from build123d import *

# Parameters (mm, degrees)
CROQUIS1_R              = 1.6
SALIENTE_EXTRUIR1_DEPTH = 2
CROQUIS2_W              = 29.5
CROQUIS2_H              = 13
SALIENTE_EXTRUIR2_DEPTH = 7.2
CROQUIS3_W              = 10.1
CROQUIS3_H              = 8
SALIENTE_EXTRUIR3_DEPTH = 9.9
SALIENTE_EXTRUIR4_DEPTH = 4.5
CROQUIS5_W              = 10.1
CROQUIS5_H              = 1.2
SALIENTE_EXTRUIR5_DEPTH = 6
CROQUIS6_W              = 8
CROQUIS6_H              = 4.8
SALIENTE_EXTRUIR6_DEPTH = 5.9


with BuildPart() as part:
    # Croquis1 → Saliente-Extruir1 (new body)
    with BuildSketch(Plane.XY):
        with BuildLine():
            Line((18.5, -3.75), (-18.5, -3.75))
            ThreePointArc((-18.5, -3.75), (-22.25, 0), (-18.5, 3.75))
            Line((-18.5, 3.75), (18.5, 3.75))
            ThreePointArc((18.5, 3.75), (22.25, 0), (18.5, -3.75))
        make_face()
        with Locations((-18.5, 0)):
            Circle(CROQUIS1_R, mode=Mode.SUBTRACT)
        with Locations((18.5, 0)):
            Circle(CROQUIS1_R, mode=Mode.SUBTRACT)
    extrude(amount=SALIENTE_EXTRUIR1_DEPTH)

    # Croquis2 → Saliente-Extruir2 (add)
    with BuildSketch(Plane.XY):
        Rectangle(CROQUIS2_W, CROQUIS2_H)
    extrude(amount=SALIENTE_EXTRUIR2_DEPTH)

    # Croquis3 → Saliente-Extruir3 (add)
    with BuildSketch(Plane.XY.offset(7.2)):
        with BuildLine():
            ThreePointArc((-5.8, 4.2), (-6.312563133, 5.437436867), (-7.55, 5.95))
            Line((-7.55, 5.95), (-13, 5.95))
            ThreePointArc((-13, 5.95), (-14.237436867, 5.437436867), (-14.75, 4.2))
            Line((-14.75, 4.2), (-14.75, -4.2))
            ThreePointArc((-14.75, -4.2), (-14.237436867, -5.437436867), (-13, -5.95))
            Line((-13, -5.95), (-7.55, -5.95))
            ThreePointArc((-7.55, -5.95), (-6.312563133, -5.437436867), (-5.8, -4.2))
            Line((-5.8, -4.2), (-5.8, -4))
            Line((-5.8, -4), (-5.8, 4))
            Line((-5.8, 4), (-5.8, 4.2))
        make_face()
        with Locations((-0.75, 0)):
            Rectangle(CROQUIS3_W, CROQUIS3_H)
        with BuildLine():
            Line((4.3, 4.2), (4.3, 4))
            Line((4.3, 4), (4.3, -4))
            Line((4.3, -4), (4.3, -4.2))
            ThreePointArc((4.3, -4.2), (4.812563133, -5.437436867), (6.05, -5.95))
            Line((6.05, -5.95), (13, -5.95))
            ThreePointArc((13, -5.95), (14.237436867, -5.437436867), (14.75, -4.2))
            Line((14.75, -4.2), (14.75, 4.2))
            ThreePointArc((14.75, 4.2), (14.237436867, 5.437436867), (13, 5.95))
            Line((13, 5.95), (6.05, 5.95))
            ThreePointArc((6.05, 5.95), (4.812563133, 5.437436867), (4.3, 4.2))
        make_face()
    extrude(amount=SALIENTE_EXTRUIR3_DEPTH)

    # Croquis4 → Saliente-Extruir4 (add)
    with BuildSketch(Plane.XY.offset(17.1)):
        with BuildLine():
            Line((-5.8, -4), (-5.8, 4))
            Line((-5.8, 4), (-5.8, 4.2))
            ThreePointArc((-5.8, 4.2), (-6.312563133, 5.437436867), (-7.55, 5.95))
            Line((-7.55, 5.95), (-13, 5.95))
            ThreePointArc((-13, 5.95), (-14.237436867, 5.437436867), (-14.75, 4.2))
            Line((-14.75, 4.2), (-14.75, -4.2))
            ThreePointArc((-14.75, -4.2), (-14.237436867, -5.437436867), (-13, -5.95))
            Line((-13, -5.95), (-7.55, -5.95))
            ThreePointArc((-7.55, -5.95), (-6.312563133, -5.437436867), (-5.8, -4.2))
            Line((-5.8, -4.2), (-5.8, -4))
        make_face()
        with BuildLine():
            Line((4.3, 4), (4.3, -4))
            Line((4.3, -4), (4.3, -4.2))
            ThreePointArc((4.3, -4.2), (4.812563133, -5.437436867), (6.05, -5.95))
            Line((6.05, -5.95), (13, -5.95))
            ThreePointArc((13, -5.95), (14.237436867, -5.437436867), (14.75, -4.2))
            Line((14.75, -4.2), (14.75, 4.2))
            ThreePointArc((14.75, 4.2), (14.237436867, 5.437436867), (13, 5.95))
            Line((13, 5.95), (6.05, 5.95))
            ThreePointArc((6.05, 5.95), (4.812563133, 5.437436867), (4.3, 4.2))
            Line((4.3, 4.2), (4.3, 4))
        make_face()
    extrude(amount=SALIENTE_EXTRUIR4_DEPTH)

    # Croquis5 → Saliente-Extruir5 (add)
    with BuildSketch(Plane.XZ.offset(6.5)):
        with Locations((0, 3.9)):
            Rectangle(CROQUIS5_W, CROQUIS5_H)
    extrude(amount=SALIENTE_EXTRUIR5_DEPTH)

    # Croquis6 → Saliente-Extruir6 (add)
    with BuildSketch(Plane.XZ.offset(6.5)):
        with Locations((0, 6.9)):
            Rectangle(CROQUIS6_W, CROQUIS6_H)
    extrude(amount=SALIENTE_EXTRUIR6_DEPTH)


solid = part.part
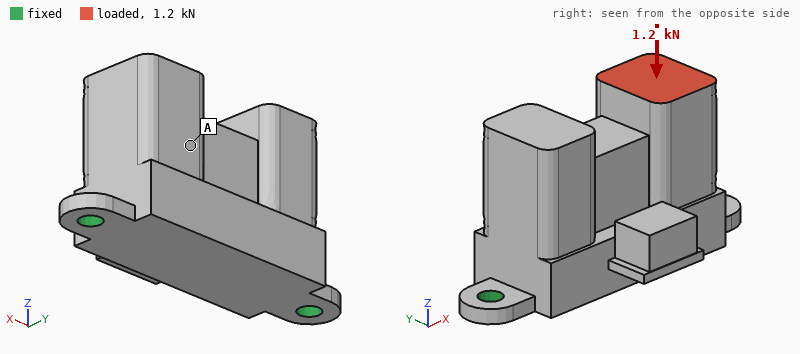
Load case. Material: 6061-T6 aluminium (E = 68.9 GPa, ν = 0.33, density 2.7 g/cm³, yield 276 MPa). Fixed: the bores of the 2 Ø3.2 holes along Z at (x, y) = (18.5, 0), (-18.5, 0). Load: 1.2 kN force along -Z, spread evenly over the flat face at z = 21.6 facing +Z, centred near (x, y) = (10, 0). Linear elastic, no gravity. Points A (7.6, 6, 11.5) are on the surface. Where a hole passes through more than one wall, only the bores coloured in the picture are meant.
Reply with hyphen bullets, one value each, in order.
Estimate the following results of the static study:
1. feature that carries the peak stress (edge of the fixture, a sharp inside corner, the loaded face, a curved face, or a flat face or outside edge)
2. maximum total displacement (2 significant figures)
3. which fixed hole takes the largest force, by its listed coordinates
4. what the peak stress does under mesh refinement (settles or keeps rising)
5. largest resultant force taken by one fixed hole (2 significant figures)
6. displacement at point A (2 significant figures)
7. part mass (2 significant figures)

- edge of the fixture
- 29 µm
- (18.5, 0)
- keeps rising
- 1.0 kN
- 21 µm
- 20 g
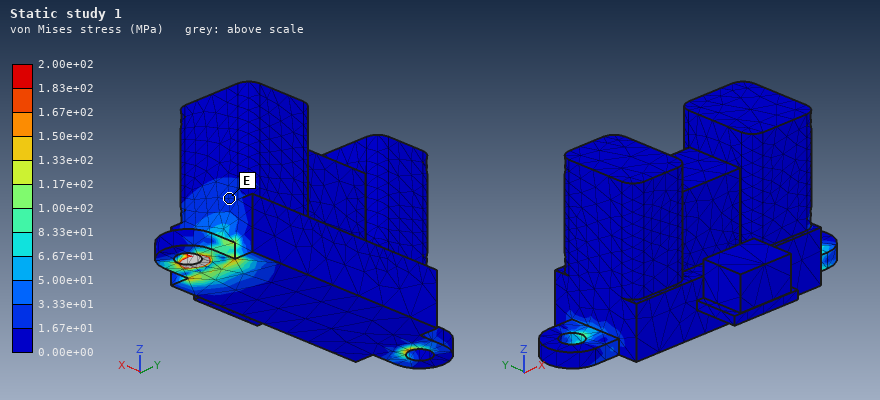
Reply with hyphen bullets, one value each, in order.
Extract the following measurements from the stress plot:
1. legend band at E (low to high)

- 1.67e+01 to 3.33e+01 MPa
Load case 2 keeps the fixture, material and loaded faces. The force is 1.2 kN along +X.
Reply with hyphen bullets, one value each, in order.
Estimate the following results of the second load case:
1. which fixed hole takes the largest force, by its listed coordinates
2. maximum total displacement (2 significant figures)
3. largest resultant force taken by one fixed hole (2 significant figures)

- (-18.5, 0)
- 45 µm
- 1.0 kN
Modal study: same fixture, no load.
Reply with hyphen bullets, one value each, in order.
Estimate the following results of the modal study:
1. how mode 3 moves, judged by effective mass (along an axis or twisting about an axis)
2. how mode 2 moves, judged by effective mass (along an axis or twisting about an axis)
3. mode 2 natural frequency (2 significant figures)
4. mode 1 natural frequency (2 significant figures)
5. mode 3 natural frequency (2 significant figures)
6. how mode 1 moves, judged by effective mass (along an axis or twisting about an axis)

- along X
- along Z
- 10000 Hz
- 2100 Hz
- 11 kHz
- along Y
